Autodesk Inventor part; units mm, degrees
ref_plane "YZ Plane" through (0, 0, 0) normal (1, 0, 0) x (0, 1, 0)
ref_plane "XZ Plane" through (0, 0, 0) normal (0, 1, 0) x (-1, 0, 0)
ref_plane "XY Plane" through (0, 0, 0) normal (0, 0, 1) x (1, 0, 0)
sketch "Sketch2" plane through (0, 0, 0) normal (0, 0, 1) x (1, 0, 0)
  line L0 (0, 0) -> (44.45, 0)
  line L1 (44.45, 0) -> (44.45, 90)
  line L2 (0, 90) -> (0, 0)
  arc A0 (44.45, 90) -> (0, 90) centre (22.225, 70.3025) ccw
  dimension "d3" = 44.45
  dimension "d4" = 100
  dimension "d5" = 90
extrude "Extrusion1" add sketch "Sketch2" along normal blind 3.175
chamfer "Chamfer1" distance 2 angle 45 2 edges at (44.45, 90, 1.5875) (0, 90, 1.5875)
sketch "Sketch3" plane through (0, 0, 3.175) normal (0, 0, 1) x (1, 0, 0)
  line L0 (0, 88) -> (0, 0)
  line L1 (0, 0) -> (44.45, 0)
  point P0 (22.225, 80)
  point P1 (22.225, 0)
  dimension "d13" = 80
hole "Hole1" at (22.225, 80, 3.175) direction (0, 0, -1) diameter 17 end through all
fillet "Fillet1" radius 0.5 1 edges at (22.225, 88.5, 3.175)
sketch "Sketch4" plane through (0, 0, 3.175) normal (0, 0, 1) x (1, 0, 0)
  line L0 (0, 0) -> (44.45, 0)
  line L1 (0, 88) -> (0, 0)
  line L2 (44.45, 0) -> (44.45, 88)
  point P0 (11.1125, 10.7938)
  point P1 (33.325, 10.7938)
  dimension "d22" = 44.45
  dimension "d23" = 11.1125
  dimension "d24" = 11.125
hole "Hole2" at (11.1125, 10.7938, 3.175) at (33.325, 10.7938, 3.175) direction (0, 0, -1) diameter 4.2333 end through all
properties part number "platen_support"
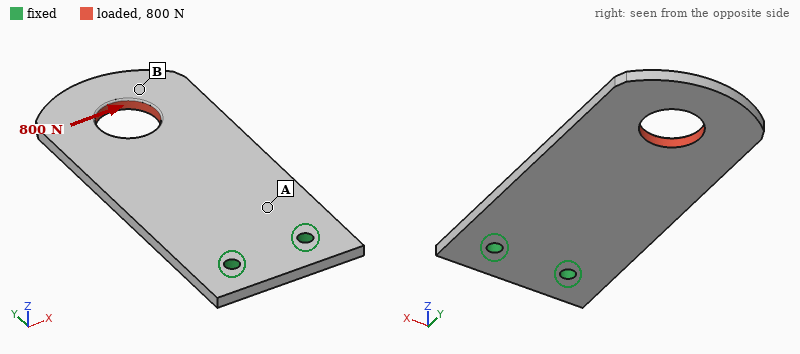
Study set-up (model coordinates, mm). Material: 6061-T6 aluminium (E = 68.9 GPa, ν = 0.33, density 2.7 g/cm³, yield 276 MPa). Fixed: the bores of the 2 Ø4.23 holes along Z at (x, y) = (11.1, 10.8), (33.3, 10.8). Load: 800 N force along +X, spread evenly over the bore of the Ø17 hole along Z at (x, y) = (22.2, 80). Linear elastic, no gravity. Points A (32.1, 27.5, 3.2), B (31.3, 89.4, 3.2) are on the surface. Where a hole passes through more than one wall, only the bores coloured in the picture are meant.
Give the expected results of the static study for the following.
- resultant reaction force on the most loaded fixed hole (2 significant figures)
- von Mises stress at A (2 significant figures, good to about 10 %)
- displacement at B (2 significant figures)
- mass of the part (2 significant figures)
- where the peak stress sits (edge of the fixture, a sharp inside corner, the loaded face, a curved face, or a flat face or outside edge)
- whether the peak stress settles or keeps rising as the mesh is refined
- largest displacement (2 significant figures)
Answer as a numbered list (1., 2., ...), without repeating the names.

1. 2.3 kN
2. 25 MPa
3. 0.12 mm
4. 35 g
5. edge of the fixture
6. keeps rising
7. 0.13 mm
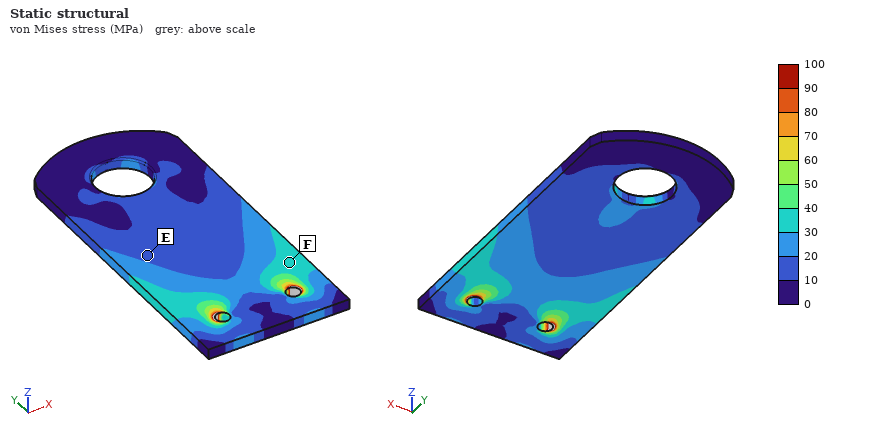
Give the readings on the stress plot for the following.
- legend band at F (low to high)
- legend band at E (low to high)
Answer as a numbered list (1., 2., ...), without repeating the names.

1. 30 to 40 MPa
2. 10 to 20 MPa
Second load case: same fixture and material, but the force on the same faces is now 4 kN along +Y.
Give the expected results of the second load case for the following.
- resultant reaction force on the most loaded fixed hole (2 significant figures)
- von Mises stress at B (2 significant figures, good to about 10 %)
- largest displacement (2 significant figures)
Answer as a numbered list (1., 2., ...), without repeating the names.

1. 2.0 kN
2. 20 MPa
3. 0.47 mm
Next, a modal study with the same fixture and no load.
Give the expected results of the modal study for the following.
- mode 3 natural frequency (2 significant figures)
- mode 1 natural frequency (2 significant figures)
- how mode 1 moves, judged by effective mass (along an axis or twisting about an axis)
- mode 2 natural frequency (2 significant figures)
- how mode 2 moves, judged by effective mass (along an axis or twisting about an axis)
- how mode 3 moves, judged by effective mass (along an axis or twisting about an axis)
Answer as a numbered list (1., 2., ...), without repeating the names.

1. 2100 Hz
2. 380 Hz
3. along Z
4. 1500 Hz
5. twisting about Y
6. along Z
